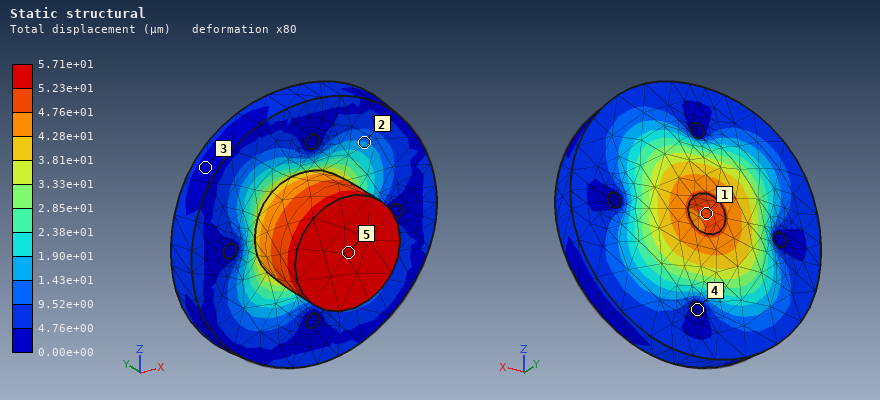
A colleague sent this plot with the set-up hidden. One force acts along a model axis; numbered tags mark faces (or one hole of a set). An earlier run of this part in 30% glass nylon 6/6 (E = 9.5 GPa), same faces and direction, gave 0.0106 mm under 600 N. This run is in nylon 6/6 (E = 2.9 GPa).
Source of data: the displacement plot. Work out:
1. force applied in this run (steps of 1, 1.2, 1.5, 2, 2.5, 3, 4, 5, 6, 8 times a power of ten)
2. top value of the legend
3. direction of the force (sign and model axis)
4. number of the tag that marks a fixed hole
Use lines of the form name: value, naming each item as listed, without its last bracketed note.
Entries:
force applied in this run: 1 kN
top value of the legend: 5.71e+01 µm
direction of the force: +Y
number of the tag that marks a fixed hole: 4
